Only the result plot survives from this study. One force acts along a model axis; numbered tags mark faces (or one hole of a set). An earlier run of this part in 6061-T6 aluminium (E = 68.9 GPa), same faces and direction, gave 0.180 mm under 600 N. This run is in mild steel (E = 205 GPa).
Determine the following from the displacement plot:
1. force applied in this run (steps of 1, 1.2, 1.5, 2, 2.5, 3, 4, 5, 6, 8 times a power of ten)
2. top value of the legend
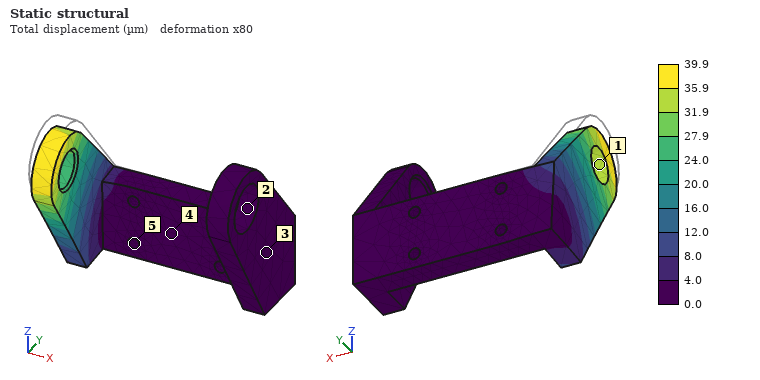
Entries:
400 N
39.9 µm
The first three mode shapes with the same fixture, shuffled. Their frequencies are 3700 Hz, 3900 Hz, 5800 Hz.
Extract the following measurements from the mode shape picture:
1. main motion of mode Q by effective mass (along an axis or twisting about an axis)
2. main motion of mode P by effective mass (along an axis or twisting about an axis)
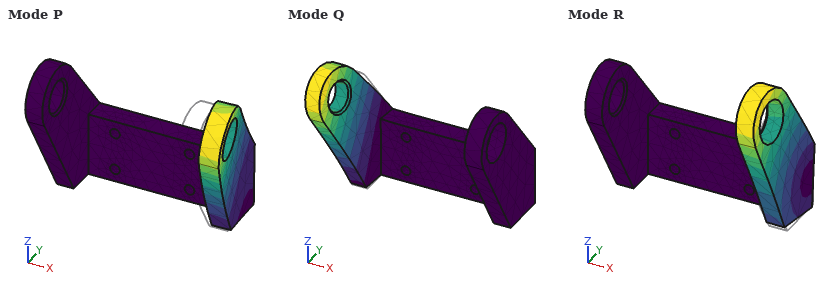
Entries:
along X
along X
